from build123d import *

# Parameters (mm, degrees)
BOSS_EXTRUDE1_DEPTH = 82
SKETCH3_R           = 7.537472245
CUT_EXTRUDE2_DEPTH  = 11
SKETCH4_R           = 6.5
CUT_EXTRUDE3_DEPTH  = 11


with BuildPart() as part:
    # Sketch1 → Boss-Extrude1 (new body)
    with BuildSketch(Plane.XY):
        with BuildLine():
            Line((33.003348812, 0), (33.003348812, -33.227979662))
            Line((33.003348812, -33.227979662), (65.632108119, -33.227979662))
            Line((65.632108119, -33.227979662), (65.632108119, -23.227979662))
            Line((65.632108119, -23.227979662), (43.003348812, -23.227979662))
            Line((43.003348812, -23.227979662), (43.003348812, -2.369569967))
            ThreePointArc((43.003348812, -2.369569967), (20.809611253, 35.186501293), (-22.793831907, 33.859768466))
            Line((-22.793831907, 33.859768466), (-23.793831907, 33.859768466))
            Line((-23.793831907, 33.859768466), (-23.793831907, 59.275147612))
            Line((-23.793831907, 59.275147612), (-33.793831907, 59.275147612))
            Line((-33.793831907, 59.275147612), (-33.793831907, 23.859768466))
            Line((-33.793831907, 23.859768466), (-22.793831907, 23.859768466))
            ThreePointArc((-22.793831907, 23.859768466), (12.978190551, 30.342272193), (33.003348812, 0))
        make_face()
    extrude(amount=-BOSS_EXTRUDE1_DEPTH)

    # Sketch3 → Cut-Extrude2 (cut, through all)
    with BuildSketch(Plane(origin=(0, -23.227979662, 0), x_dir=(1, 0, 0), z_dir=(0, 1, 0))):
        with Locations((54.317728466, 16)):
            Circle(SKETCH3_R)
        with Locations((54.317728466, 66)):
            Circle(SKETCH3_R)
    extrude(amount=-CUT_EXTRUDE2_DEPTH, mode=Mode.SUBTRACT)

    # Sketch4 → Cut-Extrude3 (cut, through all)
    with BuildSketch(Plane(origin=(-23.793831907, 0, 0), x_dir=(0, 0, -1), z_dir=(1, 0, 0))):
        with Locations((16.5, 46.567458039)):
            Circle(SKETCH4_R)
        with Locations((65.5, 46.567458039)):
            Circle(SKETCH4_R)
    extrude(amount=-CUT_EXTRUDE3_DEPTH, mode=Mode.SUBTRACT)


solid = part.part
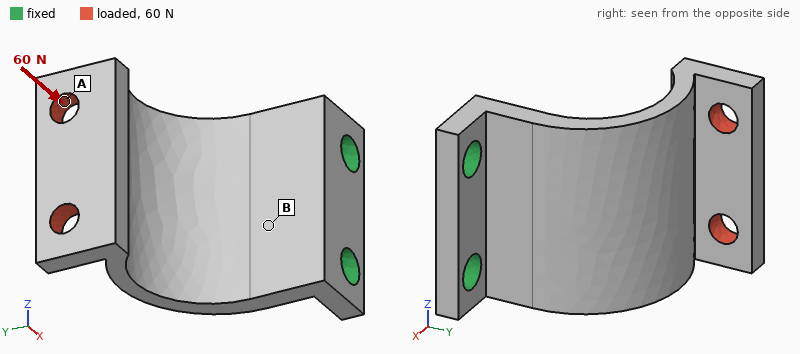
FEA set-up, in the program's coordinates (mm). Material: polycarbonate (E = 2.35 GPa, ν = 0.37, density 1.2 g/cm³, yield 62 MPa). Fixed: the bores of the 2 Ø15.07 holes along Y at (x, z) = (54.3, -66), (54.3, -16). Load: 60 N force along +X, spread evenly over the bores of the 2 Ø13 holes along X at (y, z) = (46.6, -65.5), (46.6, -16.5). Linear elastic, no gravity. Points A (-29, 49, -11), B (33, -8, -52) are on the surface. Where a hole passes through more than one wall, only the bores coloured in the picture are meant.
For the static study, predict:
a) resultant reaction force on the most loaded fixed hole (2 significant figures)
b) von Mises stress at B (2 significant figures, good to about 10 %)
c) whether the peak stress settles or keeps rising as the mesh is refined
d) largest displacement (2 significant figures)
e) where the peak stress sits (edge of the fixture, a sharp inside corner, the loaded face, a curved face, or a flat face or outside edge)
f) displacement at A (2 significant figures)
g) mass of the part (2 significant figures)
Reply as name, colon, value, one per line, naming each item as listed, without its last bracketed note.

resultant reaction force on the most loaded fixed hole: 31 N
von Mises stress at B: 2.1 MPa
whether the peak stress settles or keeps rising as the mesh is refined: keeps rising
largest displacement: 1.5 mm
where the peak stress sits: edge of the fixture
displacement at A: 1.3 mm
mass of the part: 150 g
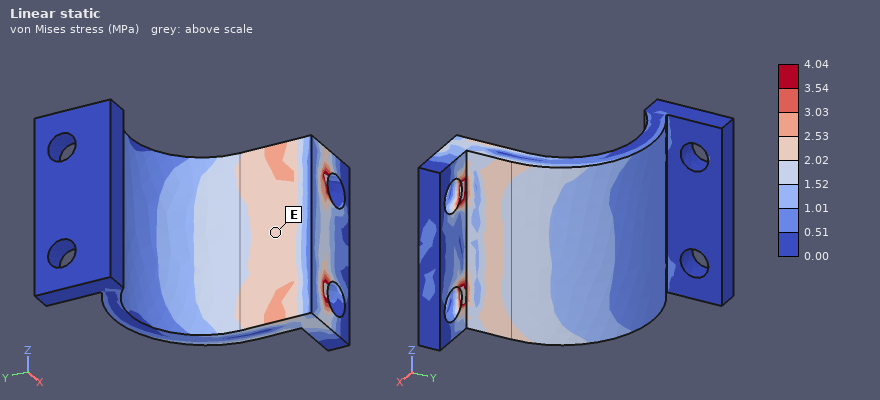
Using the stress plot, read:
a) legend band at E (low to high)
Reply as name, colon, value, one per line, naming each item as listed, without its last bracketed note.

legend band at E: 2.02 to 2.53 MPa
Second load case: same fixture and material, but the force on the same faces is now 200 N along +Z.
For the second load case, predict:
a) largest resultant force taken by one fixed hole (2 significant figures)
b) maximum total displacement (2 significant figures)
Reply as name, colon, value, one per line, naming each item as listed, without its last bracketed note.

largest resultant force taken by one fixed hole: 390 N
maximum total displacement: 1.7 mm
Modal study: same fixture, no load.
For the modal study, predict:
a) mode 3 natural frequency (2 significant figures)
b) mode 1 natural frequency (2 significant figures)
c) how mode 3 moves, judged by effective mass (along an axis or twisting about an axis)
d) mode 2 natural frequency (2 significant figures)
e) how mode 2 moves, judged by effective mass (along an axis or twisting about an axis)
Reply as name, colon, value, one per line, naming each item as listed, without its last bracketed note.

mode 3 natural frequency: 400 Hz
mode 1 natural frequency: 120 Hz
how mode 3 moves, judged by effective mass: along X
mode 2 natural frequency: 250 Hz
how mode 2 moves, judged by effective mass: along Z
